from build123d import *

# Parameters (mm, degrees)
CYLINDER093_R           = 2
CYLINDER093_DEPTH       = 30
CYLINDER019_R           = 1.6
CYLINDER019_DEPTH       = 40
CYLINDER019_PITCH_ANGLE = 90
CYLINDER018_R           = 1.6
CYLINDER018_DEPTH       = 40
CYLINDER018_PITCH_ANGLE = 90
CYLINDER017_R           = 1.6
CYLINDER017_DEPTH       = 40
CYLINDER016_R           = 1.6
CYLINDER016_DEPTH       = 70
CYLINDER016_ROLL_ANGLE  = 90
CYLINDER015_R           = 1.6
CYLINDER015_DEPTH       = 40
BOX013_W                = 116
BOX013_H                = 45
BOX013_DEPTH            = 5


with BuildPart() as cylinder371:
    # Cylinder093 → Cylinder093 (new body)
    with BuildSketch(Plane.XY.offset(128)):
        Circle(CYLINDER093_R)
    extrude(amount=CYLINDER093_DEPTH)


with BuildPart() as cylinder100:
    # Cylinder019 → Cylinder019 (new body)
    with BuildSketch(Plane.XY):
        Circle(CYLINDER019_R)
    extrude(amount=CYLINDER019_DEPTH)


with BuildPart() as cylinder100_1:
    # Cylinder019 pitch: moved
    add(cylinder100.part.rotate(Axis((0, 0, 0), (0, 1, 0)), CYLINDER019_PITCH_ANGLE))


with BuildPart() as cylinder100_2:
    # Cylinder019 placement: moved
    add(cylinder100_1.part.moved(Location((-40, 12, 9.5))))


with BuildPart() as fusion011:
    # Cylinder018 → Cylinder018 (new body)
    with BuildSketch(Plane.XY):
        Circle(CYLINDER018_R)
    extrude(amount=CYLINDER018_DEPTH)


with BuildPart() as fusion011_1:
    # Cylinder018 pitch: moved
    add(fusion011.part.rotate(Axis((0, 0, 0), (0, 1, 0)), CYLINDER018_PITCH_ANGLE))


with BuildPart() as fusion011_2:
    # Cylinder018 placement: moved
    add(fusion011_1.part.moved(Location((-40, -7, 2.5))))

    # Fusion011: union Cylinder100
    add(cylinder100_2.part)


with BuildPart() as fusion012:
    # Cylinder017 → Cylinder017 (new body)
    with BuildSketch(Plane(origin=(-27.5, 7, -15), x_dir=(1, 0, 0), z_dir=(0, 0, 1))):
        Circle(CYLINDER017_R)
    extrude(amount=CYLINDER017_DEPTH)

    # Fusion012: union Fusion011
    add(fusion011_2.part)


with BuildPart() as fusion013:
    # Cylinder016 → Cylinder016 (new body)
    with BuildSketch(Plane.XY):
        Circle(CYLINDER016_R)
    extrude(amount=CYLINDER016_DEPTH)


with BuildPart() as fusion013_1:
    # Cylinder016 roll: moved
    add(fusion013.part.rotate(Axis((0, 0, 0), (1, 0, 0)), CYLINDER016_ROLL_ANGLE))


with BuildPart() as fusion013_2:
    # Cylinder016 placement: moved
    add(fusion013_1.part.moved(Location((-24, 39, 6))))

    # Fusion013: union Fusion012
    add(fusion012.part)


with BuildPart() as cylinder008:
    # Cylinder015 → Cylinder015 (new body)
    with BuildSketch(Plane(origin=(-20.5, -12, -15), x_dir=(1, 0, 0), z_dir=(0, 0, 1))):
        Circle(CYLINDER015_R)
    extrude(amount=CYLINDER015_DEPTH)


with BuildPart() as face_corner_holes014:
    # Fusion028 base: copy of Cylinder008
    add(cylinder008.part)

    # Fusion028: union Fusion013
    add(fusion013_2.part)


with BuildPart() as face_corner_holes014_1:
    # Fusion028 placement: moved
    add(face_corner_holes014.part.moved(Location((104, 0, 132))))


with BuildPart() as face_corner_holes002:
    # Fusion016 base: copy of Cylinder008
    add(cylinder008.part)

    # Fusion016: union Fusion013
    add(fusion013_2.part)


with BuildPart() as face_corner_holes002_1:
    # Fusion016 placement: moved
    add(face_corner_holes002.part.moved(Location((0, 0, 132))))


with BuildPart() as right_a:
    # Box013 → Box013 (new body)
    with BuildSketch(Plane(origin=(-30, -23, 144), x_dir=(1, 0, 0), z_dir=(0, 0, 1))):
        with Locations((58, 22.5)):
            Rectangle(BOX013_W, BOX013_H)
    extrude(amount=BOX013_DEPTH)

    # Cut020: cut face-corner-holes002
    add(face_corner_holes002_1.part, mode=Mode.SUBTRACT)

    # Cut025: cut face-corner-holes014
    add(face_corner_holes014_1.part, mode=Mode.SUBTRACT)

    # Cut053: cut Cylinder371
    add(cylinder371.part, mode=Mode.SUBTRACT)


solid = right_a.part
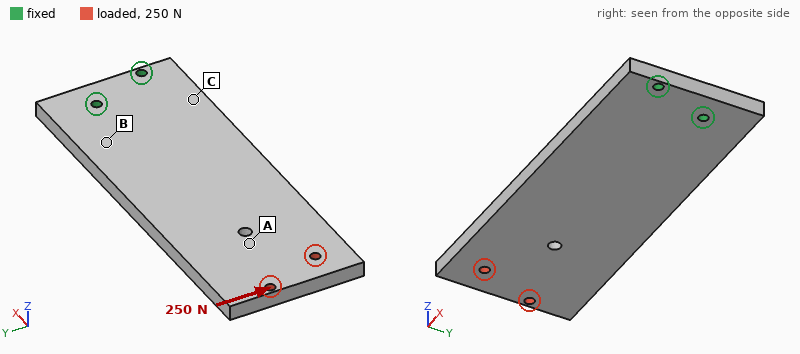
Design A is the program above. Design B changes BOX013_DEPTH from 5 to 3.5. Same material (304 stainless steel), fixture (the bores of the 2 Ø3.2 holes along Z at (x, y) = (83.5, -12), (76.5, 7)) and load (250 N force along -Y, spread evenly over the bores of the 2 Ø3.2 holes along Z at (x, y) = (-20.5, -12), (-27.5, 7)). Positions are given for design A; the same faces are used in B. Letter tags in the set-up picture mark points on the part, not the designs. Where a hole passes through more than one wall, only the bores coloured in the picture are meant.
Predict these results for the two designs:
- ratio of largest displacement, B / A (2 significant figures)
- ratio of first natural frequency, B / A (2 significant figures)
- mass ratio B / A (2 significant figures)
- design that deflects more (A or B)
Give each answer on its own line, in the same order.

1.4
0.71
0.70
B
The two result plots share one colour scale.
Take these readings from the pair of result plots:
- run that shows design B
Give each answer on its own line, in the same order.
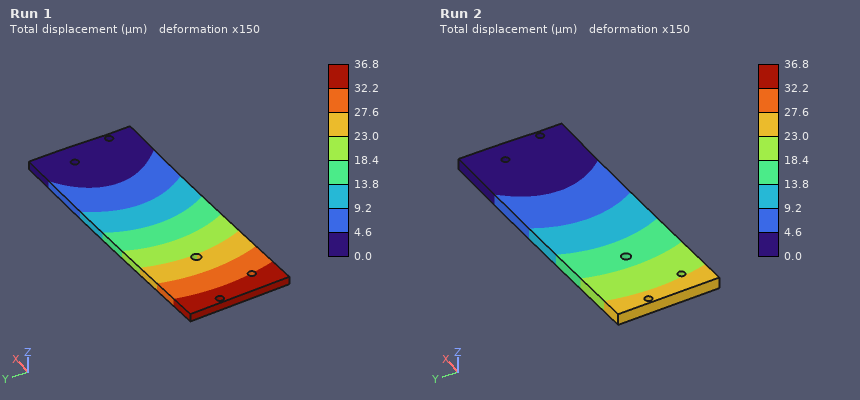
Run 1
